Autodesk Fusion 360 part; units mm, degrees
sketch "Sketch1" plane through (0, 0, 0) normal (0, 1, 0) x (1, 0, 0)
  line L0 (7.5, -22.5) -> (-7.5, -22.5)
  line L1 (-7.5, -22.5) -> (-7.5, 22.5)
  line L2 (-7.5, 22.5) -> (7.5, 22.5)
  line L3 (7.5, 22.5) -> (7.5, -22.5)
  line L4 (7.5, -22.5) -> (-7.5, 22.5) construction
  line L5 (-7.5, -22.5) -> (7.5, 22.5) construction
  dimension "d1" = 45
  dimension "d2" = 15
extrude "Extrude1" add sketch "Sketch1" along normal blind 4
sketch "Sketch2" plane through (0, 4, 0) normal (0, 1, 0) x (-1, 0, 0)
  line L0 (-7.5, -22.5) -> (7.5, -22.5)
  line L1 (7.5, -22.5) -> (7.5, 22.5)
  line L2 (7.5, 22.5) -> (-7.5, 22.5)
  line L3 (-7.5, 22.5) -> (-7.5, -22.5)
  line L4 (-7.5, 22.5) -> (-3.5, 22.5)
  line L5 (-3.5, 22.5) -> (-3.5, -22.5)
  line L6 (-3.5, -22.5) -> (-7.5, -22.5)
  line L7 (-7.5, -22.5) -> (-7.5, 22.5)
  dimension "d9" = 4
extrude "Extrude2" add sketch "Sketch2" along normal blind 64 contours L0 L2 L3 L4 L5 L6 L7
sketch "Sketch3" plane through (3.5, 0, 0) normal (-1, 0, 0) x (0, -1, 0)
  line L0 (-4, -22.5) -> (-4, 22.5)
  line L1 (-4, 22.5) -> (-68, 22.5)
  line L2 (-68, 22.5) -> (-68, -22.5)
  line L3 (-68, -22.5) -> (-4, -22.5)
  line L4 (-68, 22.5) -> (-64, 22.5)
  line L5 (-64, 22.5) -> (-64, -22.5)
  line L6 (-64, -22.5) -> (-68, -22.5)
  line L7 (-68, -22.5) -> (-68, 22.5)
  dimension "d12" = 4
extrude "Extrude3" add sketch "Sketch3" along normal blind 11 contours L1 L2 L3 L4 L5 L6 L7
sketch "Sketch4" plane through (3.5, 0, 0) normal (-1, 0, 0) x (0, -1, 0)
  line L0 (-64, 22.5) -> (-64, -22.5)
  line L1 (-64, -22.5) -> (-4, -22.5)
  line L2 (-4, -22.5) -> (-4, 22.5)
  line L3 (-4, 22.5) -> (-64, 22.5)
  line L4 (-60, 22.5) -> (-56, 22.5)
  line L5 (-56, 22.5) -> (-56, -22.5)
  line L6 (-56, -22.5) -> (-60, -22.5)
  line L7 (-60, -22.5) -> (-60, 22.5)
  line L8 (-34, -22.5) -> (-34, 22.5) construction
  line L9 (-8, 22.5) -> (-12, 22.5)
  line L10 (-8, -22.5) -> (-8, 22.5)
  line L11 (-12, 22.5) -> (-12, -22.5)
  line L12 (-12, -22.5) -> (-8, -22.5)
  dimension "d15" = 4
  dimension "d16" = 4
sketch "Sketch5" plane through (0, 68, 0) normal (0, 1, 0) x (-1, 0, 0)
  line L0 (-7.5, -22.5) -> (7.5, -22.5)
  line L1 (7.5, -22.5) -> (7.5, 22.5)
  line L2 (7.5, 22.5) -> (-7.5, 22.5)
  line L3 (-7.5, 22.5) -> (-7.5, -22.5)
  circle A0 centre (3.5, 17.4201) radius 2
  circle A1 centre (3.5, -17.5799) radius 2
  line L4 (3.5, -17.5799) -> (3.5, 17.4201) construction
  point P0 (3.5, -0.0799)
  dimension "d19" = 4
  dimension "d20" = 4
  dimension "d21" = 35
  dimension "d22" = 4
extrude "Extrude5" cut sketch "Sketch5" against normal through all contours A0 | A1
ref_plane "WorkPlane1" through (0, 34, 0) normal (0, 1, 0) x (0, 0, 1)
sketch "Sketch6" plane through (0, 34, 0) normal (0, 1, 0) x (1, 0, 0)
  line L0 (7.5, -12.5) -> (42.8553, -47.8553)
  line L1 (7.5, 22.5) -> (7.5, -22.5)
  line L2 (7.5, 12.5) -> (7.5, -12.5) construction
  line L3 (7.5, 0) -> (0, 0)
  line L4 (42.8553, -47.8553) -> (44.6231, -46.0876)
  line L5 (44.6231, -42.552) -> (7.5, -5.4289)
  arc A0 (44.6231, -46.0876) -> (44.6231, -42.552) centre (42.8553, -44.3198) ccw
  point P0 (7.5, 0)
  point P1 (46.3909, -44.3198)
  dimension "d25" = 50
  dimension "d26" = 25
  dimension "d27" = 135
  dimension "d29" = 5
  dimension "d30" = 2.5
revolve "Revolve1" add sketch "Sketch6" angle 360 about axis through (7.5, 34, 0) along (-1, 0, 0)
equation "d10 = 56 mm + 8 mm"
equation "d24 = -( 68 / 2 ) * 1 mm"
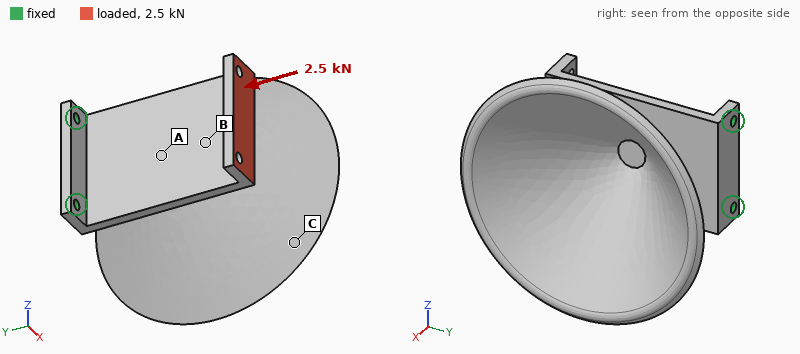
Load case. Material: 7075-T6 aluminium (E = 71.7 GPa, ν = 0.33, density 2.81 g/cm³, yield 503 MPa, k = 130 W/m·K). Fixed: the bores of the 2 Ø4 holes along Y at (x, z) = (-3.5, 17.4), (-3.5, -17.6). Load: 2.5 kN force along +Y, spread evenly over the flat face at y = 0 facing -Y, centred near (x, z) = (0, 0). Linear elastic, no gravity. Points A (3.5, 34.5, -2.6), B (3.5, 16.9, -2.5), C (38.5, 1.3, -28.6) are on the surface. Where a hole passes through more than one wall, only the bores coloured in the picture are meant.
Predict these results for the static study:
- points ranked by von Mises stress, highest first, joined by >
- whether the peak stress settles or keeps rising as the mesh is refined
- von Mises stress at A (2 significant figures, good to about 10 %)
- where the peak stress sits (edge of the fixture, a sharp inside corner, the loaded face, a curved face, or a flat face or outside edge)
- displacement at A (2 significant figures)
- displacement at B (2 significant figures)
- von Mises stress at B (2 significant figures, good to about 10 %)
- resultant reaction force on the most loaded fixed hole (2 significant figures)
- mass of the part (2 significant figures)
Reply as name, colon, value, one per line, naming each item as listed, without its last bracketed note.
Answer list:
points ranked by von Mises stress, highest first, joined by >: B > A > C
whether the peak stress settles or keeps rising as the mesh is refined: keeps rising
von Mises stress at A: 32 MPa
where the peak stress sits: edge of the fixture
displacement at A: 0.34 mm
displacement at B: 0.70 mm
von Mises stress at B: 120 MPa
resultant reaction force on the most loaded fixed hole: 1.3 kN
mass of the part: 170 g
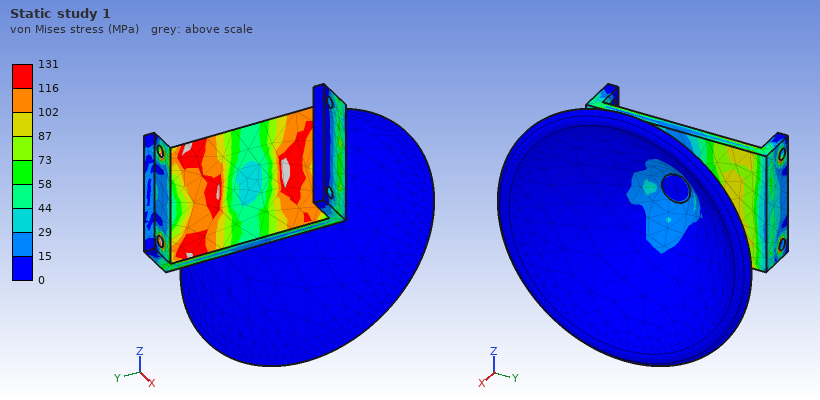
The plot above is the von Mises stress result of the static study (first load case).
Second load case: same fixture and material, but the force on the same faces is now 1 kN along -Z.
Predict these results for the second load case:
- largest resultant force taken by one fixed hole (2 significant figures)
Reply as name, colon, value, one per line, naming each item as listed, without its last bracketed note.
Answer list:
largest resultant force taken by one fixed hole: 1.9 kN
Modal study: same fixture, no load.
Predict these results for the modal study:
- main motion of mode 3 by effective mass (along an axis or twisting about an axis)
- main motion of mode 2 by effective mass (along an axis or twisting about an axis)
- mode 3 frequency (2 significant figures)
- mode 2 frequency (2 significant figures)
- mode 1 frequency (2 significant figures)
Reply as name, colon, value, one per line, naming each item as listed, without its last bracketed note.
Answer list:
main motion of mode 3 by effective mass: along Z
main motion of mode 2 by effective mass: along Z
mode 3 frequency: 1300 Hz
mode 2 frequency: 530 Hz
mode 1 frequency: 220 Hz
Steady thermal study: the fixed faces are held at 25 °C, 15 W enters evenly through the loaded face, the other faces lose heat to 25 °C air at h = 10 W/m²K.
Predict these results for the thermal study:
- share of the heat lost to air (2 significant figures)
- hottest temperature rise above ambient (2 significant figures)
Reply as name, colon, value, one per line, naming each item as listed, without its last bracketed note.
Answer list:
share of the heat lost to air: 32 %
hottest temperature rise above ambient: 38 K
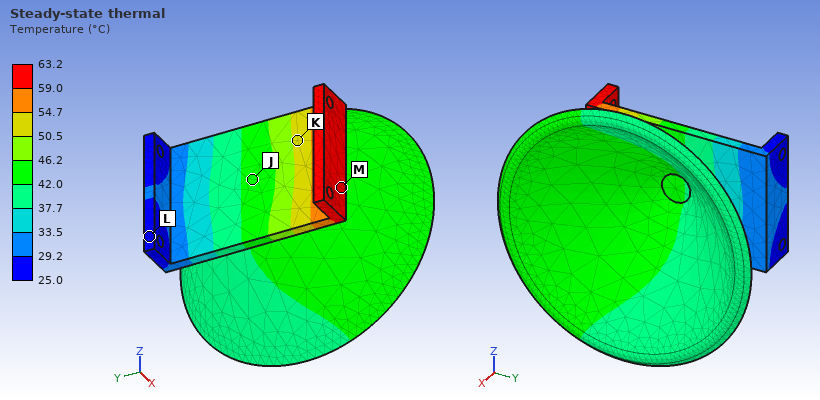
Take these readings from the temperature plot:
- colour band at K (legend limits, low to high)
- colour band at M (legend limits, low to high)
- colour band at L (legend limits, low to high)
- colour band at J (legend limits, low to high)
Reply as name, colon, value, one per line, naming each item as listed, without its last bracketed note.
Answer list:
colour band at K: 50.5 to 54.7 °C
colour band at M: 59.0 to 63.2 °C
colour band at L: 25.0 to 29.2 °C
colour band at J: 42.0 to 46.2 °C
